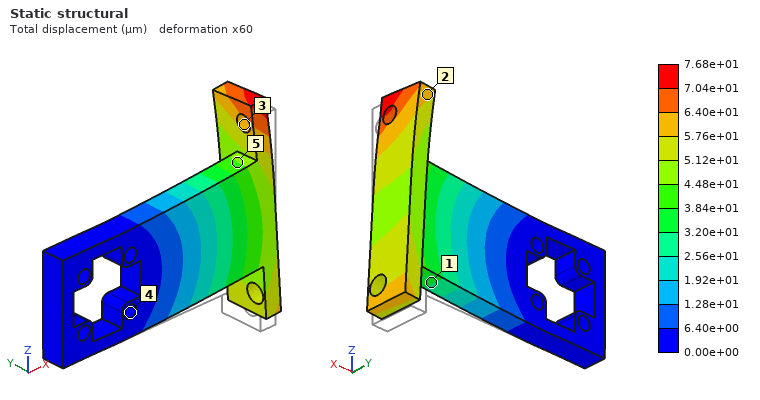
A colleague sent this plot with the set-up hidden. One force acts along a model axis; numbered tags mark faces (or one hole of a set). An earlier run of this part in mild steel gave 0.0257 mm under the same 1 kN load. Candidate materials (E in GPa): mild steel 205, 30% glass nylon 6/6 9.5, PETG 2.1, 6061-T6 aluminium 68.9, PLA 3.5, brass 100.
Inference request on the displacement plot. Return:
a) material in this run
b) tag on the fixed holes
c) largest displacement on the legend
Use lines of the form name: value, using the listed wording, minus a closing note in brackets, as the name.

material in this run: 6061-T6 aluminium
tag on the fixed holes: 4
largest displacement on the legend: 7.68e+01 µm
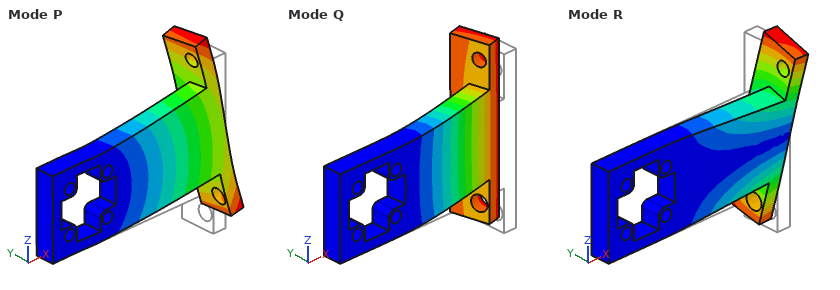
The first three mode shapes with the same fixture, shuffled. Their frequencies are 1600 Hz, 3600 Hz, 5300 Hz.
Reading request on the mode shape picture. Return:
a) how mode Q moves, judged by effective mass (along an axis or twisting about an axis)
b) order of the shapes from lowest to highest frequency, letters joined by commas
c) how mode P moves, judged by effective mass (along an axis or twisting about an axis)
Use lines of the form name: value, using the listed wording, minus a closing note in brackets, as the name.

how mode Q moves, judged by effective mass: along Y
order of the shapes from lowest to highest frequency, letters joined by commas: Q, R, P
how mode P moves, judged by effective mass: along Z
